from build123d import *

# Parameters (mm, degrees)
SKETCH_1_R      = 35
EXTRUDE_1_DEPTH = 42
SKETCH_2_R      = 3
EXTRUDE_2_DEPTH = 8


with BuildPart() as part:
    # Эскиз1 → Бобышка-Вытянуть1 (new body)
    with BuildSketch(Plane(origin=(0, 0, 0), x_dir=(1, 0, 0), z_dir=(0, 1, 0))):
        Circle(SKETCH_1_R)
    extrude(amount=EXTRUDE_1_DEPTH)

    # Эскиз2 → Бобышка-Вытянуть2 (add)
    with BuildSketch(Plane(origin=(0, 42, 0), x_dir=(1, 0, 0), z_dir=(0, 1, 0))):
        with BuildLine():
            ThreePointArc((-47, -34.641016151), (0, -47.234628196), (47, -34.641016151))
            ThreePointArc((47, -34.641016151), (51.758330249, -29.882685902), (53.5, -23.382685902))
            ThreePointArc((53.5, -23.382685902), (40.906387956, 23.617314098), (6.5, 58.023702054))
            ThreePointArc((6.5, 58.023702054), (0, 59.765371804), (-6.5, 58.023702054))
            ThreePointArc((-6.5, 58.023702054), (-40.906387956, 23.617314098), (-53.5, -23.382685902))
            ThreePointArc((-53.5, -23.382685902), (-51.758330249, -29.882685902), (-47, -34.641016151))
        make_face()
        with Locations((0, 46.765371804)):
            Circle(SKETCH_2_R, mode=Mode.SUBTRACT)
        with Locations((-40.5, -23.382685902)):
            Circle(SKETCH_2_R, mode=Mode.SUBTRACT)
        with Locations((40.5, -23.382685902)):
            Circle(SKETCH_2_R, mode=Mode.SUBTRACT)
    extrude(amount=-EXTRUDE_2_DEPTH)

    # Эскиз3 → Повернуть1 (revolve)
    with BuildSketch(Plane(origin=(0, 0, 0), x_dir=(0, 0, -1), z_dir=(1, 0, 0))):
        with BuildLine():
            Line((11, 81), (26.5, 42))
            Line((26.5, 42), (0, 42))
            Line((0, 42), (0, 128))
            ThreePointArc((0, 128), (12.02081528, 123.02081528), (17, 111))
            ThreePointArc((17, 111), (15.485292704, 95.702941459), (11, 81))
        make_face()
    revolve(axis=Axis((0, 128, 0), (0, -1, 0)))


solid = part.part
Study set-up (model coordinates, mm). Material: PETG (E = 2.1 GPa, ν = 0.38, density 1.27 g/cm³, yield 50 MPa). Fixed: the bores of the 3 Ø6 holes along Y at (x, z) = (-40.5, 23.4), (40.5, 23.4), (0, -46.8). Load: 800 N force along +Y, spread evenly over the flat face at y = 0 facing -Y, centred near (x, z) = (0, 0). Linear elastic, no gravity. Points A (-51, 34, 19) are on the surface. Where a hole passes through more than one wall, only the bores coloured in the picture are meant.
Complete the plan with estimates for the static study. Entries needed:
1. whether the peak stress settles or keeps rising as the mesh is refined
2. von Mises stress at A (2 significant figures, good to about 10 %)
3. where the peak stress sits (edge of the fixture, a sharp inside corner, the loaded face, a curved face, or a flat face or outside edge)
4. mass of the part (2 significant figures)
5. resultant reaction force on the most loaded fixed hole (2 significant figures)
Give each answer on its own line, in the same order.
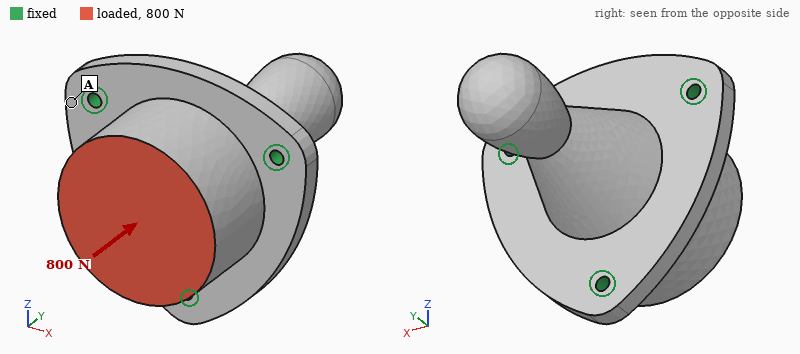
keeps rising
1.0 MPa
edge of the fixture
350 g
280 N
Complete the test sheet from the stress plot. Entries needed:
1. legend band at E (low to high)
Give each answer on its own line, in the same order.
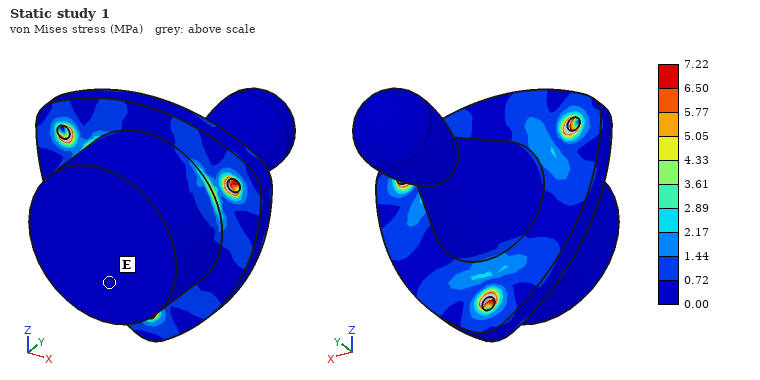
0.00 to 0.72 MPa
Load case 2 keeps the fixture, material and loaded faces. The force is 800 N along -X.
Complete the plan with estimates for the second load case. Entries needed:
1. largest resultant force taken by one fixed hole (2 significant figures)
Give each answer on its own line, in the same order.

530 N
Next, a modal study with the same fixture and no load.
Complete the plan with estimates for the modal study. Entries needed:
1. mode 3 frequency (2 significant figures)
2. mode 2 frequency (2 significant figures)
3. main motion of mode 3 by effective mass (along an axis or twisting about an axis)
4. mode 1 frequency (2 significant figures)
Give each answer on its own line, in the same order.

950 Hz
640 Hz
along Y
640 Hz
